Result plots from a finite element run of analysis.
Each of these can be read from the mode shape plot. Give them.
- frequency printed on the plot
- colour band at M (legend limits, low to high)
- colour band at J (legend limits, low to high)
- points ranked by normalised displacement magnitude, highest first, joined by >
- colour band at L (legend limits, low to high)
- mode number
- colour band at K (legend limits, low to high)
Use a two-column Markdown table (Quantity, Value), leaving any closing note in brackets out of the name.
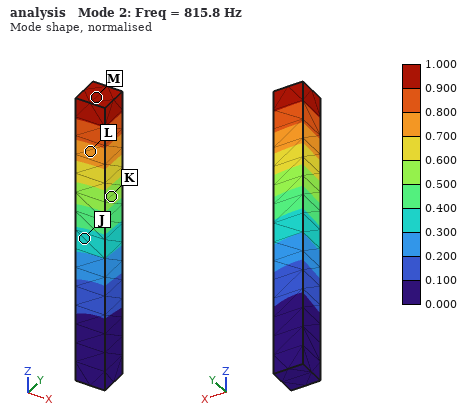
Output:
| Quantity | Value |
|---|---|
| frequency printed on the plot | 815.8 Hz |
| colour band at M | 0.900 to 1.000 |
| colour band at J | 0.300 to 0.400 |
| points ranked by normalised displacement magnitude, highest first, joined by > | M > L > K > J |
| colour band at L | 0.700 to 0.800 |
| mode number | 2 |
| colour band at K | 0.500 to 0.600 |
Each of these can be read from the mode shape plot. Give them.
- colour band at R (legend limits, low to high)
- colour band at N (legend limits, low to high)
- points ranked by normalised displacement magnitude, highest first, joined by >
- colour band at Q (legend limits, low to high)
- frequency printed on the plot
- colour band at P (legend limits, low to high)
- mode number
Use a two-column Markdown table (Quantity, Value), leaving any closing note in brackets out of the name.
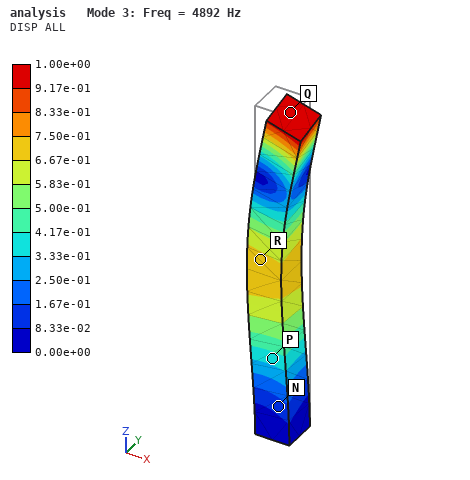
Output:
| Quantity | Value |
|---|---|
| colour band at R | 6.67e-01 to 7.50e-01 |
| colour band at N | 8.33e-02 to 1.67e-01 |
| points ranked by normalised displacement magnitude, highest first, joined by > | Q > R > P > N |
| colour band at Q | 9.17e-01 to 1.00e+00 |
| frequency printed on the plot | 4892 Hz |
| colour band at P | 3.33e-01 to 4.17e-01 |
| mode number | 3 |
